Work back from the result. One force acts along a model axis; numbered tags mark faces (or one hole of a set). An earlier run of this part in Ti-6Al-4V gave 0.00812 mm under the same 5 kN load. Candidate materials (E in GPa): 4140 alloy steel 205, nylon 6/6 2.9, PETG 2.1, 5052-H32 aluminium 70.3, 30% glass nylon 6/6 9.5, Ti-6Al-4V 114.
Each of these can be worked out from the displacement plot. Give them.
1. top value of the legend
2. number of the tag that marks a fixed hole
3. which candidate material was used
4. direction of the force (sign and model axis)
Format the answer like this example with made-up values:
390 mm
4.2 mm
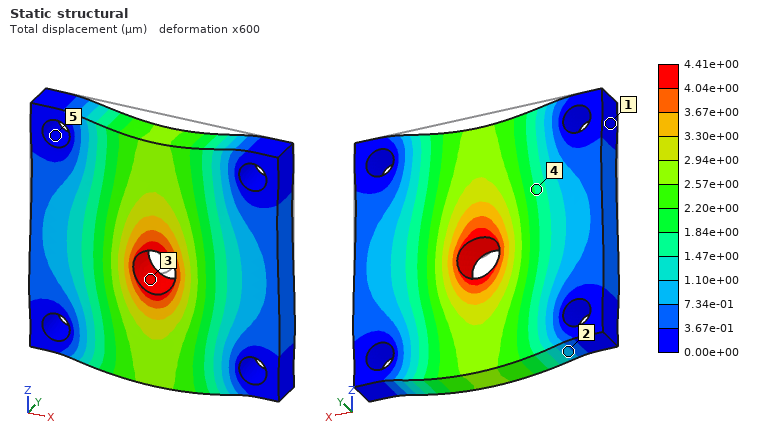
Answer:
4.41e+00 µm
5
4140 alloy steel
-Z
